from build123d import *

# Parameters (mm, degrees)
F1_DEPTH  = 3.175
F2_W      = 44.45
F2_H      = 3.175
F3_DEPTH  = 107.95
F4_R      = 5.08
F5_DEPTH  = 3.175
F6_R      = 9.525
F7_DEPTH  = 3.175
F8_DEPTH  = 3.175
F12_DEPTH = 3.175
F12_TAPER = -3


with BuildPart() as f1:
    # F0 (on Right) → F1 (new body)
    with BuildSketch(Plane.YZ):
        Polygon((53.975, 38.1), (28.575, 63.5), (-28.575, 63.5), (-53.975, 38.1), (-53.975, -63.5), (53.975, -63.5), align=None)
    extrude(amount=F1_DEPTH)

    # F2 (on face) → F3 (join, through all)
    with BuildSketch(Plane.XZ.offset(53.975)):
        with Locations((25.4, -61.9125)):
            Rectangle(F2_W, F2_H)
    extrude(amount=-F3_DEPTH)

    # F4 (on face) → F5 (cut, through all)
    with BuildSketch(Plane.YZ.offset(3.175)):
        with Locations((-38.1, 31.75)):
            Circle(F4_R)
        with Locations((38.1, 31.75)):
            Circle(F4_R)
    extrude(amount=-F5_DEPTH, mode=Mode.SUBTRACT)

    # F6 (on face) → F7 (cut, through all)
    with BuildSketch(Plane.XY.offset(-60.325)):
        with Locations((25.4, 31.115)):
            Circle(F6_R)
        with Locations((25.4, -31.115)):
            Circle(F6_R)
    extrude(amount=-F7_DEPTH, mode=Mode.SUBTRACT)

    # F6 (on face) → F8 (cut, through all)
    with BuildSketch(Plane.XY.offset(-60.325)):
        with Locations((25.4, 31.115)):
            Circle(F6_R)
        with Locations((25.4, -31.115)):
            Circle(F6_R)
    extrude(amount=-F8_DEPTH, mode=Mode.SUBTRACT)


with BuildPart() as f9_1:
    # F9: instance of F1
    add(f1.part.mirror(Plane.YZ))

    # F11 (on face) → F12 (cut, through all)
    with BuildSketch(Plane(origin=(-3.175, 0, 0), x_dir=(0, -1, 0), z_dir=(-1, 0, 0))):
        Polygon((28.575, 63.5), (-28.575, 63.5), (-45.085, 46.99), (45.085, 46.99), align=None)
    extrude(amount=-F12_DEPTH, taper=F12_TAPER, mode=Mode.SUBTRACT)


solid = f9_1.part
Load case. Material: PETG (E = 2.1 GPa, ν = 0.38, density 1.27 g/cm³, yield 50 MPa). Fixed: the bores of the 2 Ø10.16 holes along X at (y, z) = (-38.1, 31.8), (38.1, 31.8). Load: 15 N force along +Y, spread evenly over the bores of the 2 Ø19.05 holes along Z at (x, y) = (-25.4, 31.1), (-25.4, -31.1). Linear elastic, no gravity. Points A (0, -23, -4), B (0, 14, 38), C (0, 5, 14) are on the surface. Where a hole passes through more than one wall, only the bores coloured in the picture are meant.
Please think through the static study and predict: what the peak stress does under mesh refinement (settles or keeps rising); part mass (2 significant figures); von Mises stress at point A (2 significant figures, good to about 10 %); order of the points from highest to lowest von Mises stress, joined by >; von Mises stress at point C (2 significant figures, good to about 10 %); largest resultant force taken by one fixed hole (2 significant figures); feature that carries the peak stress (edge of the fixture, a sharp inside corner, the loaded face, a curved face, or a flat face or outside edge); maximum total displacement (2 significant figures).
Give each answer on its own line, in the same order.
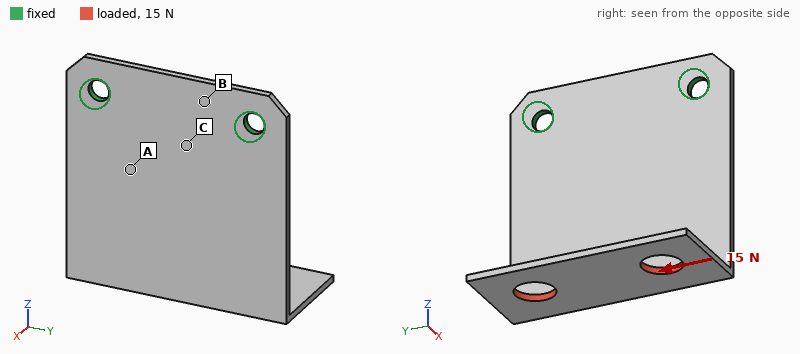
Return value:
keeps rising
64 g
1.1 MPa
A > C > B
0.58 MPa
19 N
edge of the fixture
1.6 mm
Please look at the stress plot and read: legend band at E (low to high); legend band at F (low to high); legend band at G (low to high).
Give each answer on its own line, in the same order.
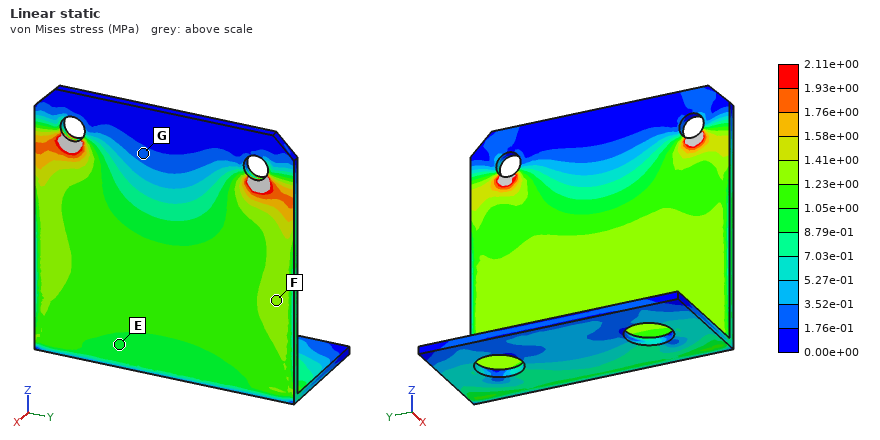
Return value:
8.79e-01 to 1.05e+00 MPa
1.23e+00 to 1.41e+00 MPa
1.76e-01 to 3.52e-01 MPa
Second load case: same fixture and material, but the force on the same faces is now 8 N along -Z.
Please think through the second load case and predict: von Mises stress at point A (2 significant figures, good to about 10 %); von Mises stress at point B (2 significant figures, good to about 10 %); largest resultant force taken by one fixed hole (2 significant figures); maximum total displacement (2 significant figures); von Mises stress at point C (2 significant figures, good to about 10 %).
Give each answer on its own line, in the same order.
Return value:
0.91 MPa
0.35 MPa
4.1 N
1.9 mm
0.77 MPa
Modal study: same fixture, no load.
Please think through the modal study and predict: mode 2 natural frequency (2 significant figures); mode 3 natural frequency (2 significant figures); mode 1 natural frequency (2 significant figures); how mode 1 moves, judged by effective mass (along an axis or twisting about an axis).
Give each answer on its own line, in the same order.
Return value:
99 Hz
180 Hz
44 Hz
along X
